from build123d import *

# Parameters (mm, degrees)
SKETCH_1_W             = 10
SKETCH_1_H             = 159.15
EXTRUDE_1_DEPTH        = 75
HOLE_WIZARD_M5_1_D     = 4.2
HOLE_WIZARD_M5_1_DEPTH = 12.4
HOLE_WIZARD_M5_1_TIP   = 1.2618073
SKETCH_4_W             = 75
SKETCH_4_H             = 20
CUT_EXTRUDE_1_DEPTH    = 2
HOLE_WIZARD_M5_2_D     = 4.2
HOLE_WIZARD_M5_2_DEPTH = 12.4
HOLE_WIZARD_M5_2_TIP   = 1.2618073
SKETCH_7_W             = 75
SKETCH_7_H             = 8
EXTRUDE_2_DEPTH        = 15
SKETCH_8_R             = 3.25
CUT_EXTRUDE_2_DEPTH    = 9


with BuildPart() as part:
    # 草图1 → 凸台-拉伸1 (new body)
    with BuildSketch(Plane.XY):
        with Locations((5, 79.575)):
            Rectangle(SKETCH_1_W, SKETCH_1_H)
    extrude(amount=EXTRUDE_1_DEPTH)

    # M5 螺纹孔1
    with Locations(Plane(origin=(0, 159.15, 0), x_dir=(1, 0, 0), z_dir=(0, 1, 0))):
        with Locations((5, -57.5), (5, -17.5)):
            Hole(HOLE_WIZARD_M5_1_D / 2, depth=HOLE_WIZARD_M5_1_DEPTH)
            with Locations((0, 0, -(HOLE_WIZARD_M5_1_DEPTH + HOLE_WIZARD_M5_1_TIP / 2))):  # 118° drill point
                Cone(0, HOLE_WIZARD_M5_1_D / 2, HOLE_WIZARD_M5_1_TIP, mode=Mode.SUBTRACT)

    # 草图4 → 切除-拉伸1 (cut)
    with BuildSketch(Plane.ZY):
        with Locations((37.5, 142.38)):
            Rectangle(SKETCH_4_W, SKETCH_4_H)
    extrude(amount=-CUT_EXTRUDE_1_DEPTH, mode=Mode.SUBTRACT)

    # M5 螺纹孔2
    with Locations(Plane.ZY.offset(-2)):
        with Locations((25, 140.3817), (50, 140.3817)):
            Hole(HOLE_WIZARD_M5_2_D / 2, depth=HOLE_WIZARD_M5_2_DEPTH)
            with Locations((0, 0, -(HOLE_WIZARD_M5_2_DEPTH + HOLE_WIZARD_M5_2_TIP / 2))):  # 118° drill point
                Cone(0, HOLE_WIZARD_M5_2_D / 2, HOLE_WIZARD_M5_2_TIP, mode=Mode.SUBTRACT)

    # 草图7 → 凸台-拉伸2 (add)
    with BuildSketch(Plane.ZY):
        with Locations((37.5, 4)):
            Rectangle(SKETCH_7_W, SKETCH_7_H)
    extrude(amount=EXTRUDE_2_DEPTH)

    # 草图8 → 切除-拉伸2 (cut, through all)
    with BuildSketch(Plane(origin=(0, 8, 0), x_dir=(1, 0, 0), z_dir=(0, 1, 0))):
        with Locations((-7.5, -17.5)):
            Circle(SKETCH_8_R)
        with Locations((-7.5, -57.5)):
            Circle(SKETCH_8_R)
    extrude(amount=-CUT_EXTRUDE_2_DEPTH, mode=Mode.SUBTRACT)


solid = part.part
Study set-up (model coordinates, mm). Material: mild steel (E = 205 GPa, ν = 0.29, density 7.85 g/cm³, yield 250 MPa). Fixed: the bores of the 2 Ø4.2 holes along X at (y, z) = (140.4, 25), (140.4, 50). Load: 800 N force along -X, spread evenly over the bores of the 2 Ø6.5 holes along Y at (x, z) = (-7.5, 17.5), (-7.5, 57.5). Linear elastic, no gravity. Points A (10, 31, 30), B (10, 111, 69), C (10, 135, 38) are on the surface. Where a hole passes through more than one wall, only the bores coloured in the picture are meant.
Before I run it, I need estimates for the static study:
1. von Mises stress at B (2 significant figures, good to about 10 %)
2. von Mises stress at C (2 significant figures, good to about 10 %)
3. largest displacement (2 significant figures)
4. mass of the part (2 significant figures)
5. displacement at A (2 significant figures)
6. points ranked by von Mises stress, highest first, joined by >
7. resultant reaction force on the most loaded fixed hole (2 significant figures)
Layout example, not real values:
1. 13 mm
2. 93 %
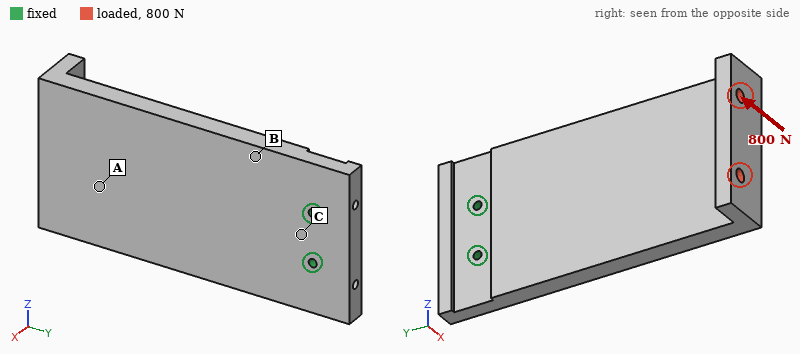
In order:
1. 67 MPa
2. 110 MPa
3. 0.77 mm
4. 980 g
5. 0.53 mm
6. C > B > A
7. 440 N
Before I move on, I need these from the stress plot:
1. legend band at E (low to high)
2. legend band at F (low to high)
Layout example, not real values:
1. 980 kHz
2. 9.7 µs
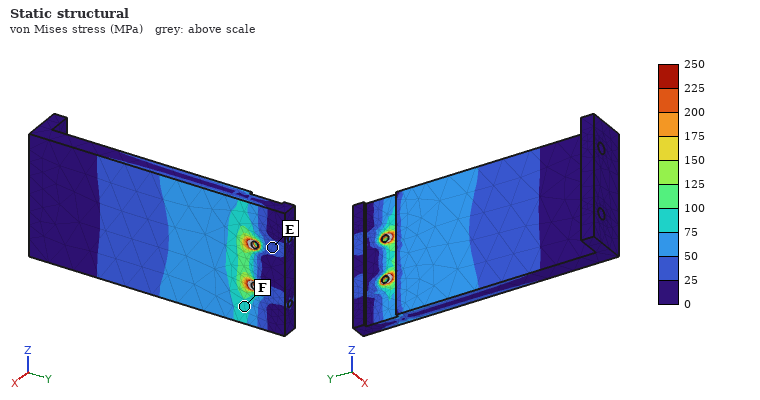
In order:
1. 25 to 50 MPa
2. 75 to 100 MPa
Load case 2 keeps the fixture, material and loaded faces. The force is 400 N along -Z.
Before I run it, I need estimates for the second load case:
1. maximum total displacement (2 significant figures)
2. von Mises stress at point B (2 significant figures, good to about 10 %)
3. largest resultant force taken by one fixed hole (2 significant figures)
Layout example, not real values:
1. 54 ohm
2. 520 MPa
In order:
1. 25 µm
2. 5.0 MPa
3. 2.0 kN
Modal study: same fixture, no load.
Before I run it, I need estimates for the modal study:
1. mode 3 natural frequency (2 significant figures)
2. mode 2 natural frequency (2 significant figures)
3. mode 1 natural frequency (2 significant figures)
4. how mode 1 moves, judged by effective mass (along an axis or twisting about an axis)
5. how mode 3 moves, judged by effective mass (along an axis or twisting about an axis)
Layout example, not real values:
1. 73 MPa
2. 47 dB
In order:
1. 1400 Hz
2. 1300 Hz
3. 300 Hz
4. along X
5. along Z
